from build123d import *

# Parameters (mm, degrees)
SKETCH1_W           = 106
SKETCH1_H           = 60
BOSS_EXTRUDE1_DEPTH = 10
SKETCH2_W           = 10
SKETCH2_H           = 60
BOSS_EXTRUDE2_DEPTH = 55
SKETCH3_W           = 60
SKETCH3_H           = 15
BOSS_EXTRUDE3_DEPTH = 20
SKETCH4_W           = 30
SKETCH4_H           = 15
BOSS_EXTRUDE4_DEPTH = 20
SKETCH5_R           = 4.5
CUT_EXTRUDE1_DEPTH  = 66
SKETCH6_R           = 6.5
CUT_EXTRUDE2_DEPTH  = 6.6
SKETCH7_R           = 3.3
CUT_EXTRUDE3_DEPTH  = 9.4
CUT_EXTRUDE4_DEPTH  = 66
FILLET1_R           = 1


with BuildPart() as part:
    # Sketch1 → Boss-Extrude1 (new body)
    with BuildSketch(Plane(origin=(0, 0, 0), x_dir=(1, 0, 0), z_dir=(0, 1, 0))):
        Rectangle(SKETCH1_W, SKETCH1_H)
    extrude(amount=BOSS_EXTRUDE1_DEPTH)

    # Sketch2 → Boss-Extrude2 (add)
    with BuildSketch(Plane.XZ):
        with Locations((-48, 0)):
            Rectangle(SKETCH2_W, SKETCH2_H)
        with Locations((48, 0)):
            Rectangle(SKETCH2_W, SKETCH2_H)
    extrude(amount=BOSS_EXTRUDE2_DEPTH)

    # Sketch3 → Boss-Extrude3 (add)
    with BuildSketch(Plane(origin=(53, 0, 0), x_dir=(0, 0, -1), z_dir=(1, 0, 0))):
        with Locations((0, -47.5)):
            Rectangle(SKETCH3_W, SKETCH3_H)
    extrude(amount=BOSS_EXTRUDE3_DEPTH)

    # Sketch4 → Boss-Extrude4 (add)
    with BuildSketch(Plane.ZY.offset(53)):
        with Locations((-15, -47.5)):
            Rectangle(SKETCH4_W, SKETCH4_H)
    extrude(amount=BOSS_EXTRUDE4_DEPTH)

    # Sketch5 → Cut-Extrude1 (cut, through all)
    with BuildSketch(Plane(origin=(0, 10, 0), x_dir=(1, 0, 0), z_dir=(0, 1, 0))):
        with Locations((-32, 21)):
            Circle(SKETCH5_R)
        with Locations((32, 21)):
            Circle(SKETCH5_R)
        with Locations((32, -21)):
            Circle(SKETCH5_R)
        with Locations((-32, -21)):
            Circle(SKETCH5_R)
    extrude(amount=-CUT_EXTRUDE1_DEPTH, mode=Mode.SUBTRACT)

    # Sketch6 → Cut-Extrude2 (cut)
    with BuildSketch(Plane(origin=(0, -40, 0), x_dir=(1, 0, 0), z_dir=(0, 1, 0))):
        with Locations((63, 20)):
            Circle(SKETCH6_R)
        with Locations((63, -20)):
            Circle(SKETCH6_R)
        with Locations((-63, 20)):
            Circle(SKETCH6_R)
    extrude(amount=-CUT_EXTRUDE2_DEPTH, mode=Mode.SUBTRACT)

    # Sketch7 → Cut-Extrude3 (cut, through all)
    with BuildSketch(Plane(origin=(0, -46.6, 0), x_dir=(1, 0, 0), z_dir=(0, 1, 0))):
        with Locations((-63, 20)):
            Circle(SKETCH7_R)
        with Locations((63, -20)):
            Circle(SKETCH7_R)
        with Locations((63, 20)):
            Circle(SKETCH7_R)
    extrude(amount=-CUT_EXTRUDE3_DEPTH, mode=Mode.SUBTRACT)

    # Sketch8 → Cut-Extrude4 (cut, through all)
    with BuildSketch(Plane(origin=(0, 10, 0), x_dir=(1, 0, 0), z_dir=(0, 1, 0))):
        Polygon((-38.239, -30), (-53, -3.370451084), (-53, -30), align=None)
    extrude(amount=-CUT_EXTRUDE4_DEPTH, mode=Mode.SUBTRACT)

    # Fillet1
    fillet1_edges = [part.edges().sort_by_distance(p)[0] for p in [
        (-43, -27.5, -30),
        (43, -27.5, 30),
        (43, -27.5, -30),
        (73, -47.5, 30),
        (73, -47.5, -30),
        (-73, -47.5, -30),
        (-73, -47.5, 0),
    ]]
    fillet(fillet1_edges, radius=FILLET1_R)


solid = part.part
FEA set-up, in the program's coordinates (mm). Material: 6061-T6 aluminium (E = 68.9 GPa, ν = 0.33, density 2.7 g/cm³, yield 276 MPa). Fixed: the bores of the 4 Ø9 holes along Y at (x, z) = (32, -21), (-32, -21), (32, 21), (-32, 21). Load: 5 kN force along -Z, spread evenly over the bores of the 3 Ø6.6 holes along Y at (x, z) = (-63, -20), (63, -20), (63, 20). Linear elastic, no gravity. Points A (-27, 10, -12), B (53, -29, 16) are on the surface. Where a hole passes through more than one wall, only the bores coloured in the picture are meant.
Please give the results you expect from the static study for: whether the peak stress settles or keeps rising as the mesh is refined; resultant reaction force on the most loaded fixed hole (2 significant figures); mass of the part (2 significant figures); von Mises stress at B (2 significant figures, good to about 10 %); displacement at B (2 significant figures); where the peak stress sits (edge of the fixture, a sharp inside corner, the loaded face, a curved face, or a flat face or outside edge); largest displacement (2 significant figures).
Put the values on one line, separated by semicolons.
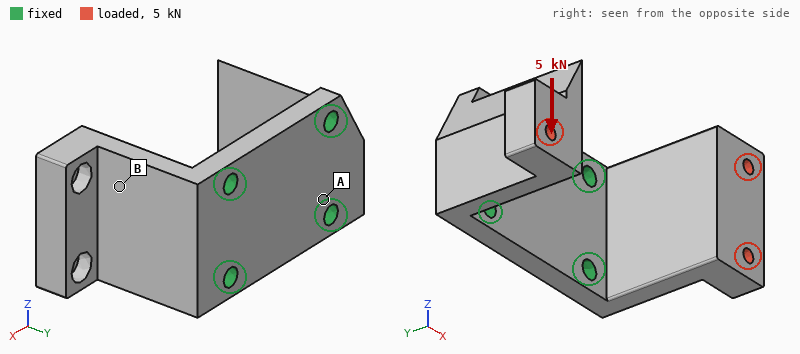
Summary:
keeps rising; 4.9 kN; 370 g; 40 MPa; 0.053 mm; a sharp inside corner; 0.15 mm
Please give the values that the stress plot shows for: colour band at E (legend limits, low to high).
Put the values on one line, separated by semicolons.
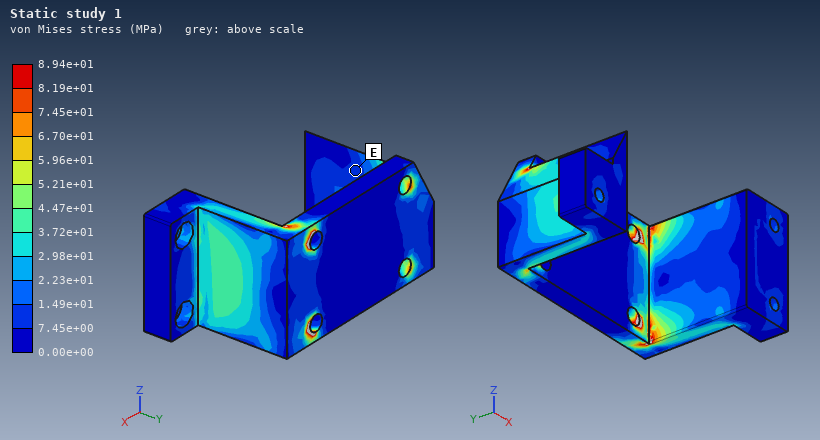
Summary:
7.45e+00 to 1.49e+01 MPa
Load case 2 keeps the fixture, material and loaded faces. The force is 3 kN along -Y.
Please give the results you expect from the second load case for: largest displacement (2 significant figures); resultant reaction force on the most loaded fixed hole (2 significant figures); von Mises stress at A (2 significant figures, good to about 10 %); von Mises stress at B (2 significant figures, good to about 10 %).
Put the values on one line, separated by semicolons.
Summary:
0.30 mm; 1.0 kN; 6.2 MPa; 31 MPa
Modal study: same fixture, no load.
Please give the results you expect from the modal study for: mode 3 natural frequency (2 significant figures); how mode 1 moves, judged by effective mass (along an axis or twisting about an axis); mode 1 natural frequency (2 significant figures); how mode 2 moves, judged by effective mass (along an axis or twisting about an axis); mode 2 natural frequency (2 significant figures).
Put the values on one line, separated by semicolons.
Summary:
3300 Hz; along X; 1100 Hz; along X; 1200 Hz
